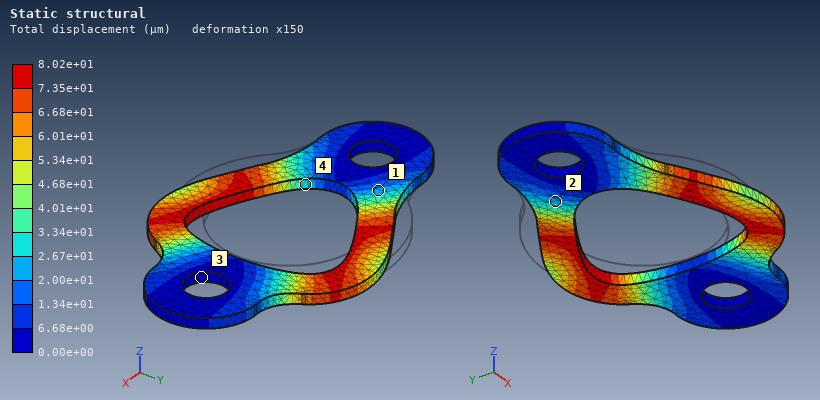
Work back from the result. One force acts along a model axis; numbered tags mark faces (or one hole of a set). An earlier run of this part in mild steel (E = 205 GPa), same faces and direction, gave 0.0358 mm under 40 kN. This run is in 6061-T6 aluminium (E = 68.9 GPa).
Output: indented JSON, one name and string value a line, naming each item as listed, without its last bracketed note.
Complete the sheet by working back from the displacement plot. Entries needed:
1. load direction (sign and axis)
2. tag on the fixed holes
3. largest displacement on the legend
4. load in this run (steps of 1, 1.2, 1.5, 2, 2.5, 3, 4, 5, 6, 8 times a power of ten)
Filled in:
{
  "load direction": "+X",
  "tag on the fixed holes": "3",
  "largest displacement on the legend": "8.02e+01 µm",
  "load in this run": "30 kN"
}
